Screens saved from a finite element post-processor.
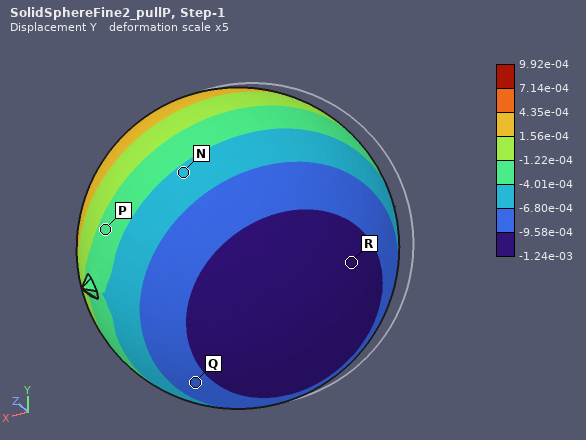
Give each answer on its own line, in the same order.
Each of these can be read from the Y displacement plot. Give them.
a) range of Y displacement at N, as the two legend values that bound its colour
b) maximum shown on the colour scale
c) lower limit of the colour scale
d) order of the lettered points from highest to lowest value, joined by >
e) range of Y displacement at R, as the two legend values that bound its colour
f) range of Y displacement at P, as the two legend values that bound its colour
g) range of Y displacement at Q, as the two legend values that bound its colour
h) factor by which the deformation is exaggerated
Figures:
-6.80e-04 to -4.01e-04
9.92e-04
-1.24e-03
P > N > Q > R
-1.24e-03 to -9.58e-04
-4.01e-04 to -1.22e-04
-9.58e-04 to -6.80e-04
5
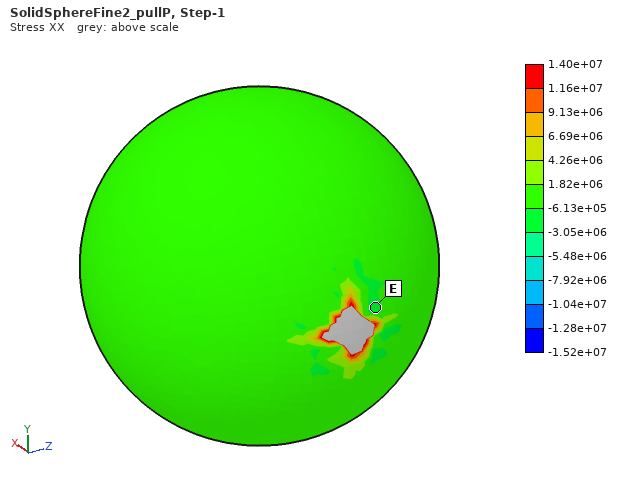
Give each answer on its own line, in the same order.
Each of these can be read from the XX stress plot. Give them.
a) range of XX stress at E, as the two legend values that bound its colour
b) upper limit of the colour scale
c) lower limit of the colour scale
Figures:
-3.05e+06 to -6.13e+05
1.40e+07
-1.52e+07
